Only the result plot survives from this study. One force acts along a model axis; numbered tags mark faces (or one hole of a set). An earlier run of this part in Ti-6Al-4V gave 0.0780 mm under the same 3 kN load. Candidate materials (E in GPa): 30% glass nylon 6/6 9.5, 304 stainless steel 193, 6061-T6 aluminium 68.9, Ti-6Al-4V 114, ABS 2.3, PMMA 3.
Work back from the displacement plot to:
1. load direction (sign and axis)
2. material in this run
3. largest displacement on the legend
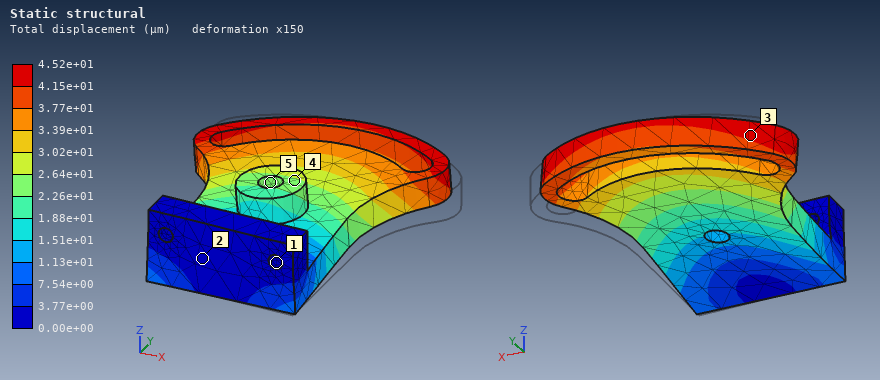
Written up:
-X
304 stainless steel
4.52e+01 µm
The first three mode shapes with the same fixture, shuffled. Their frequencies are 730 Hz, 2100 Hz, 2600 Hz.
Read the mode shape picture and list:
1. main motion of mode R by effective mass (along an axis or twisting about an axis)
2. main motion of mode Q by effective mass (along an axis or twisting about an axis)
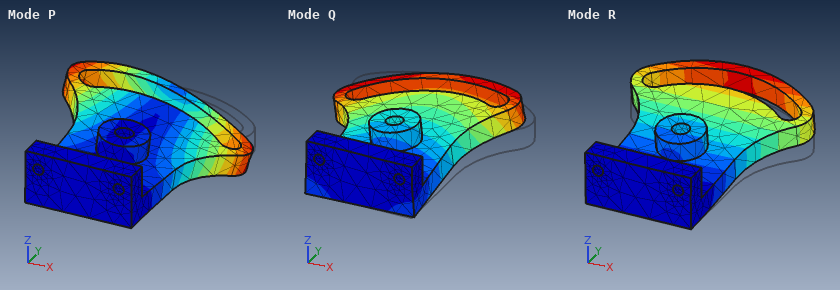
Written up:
along Z
along X
